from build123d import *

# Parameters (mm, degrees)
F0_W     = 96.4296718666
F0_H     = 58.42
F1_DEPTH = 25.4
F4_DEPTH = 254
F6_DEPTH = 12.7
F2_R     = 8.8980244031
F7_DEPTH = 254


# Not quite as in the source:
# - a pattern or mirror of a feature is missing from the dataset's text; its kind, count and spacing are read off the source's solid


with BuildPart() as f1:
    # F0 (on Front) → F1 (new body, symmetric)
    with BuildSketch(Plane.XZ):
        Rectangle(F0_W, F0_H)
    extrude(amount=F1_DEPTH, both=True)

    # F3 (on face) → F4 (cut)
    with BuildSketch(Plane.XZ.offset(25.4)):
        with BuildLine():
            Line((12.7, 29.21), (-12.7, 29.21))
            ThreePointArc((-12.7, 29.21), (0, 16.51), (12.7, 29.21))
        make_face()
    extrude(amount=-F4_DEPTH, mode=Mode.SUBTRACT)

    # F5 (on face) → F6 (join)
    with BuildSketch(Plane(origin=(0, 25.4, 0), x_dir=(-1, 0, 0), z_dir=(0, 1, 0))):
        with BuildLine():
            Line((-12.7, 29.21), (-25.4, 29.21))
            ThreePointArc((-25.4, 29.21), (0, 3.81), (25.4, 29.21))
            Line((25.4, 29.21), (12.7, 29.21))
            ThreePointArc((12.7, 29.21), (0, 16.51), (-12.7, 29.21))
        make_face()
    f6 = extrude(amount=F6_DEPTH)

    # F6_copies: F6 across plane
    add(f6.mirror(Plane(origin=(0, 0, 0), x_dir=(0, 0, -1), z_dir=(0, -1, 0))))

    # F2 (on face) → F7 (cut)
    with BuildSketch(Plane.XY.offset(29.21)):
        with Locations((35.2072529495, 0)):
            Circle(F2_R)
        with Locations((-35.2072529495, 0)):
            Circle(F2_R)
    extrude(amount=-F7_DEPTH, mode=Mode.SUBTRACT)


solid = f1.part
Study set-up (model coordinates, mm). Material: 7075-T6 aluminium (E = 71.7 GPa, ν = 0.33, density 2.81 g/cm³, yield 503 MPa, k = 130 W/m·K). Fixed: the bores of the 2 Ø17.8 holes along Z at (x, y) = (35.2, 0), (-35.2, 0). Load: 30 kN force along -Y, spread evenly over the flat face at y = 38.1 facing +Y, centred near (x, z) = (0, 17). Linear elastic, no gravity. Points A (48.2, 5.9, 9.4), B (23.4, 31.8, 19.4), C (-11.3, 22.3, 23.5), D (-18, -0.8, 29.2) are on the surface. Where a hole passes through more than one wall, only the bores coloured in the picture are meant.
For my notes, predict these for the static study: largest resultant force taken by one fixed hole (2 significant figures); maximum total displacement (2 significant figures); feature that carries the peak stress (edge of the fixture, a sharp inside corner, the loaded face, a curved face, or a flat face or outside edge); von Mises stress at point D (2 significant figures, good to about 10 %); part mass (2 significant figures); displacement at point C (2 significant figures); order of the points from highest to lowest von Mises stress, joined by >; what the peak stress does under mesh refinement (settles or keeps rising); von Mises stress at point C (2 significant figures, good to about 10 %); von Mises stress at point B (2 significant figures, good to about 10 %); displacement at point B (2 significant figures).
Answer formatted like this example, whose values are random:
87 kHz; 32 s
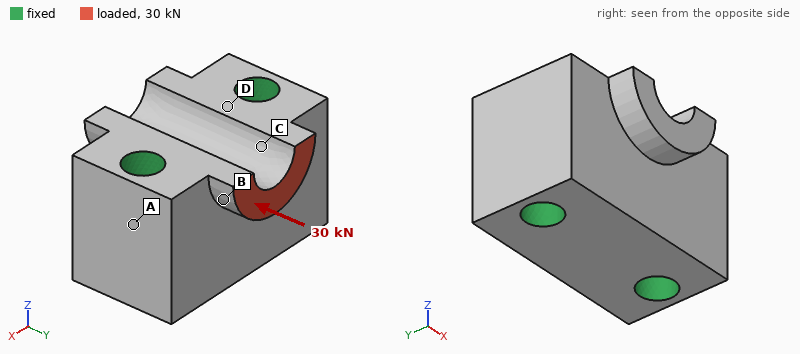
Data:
16 kN; 26 µm; a sharp inside corner; 16 MPa; 740 g; 14 µm; B > C > D > A; keeps rising; 29 MPa; 45 MPa; 17 µm
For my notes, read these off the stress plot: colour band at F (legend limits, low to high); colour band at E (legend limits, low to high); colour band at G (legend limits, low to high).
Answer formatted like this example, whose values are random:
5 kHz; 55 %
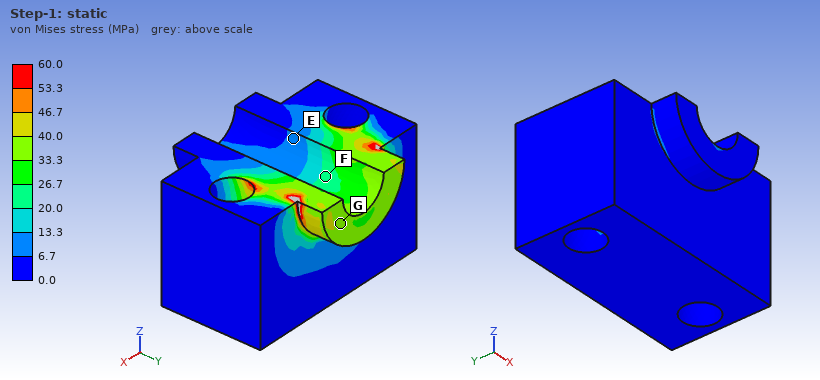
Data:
20.0 to 26.7 MPa; 6.7 to 13.3 MPa; 33.3 to 40.0 MPa
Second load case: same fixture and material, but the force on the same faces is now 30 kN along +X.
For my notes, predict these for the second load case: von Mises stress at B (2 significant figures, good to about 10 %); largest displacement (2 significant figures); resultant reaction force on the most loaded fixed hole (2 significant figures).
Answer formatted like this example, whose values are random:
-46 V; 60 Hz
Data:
100 MPa; 88 µm; 21 kN
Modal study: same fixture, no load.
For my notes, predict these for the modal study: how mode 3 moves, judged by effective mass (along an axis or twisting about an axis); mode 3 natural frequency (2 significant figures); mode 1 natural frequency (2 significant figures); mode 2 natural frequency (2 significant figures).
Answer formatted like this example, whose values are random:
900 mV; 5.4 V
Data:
along Y; 20 kHz; 19 kHz; 19 kHz
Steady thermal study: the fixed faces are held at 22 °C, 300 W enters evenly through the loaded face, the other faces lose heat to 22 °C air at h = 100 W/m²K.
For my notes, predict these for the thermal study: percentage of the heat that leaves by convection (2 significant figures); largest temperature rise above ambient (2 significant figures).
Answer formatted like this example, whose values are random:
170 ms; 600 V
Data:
6.2 %; 72 K
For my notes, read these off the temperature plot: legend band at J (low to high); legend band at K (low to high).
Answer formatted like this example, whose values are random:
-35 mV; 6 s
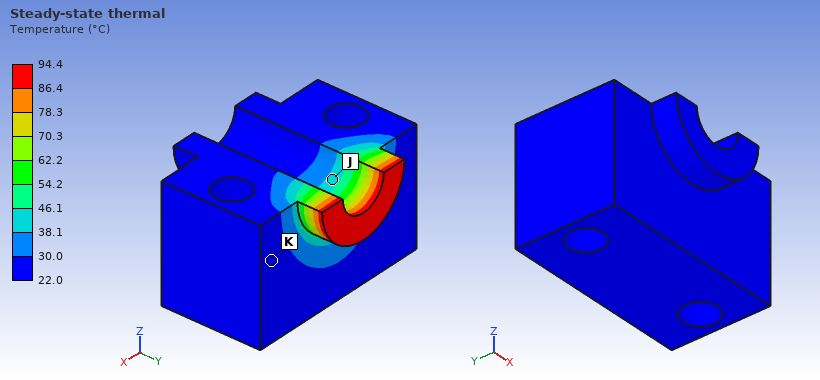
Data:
38.1 to 46.1 °C; 22.0 to 30.0 °C
